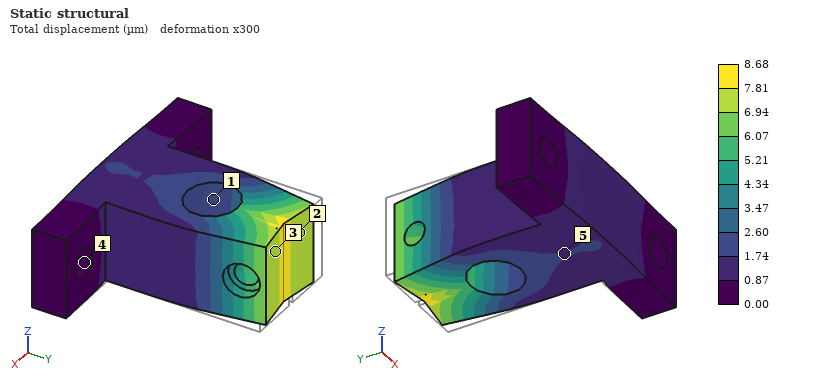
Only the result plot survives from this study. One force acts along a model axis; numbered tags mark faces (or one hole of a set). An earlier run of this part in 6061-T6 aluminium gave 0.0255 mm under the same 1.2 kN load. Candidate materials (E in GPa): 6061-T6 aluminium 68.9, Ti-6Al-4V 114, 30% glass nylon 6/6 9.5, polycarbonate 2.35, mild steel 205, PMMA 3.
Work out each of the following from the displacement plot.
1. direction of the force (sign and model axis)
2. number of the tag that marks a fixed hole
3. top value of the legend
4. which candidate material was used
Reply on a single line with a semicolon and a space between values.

-Y; 4; 8.68 µm; mild steel
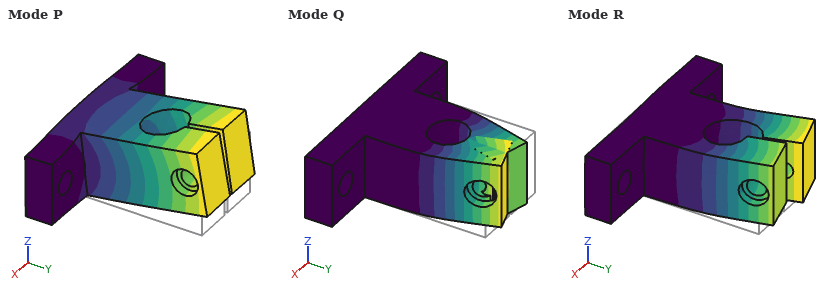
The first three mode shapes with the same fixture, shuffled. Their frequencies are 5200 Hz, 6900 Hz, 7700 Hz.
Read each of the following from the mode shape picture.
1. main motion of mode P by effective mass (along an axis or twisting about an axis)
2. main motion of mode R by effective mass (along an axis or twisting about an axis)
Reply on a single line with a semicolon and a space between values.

along Z; along X
